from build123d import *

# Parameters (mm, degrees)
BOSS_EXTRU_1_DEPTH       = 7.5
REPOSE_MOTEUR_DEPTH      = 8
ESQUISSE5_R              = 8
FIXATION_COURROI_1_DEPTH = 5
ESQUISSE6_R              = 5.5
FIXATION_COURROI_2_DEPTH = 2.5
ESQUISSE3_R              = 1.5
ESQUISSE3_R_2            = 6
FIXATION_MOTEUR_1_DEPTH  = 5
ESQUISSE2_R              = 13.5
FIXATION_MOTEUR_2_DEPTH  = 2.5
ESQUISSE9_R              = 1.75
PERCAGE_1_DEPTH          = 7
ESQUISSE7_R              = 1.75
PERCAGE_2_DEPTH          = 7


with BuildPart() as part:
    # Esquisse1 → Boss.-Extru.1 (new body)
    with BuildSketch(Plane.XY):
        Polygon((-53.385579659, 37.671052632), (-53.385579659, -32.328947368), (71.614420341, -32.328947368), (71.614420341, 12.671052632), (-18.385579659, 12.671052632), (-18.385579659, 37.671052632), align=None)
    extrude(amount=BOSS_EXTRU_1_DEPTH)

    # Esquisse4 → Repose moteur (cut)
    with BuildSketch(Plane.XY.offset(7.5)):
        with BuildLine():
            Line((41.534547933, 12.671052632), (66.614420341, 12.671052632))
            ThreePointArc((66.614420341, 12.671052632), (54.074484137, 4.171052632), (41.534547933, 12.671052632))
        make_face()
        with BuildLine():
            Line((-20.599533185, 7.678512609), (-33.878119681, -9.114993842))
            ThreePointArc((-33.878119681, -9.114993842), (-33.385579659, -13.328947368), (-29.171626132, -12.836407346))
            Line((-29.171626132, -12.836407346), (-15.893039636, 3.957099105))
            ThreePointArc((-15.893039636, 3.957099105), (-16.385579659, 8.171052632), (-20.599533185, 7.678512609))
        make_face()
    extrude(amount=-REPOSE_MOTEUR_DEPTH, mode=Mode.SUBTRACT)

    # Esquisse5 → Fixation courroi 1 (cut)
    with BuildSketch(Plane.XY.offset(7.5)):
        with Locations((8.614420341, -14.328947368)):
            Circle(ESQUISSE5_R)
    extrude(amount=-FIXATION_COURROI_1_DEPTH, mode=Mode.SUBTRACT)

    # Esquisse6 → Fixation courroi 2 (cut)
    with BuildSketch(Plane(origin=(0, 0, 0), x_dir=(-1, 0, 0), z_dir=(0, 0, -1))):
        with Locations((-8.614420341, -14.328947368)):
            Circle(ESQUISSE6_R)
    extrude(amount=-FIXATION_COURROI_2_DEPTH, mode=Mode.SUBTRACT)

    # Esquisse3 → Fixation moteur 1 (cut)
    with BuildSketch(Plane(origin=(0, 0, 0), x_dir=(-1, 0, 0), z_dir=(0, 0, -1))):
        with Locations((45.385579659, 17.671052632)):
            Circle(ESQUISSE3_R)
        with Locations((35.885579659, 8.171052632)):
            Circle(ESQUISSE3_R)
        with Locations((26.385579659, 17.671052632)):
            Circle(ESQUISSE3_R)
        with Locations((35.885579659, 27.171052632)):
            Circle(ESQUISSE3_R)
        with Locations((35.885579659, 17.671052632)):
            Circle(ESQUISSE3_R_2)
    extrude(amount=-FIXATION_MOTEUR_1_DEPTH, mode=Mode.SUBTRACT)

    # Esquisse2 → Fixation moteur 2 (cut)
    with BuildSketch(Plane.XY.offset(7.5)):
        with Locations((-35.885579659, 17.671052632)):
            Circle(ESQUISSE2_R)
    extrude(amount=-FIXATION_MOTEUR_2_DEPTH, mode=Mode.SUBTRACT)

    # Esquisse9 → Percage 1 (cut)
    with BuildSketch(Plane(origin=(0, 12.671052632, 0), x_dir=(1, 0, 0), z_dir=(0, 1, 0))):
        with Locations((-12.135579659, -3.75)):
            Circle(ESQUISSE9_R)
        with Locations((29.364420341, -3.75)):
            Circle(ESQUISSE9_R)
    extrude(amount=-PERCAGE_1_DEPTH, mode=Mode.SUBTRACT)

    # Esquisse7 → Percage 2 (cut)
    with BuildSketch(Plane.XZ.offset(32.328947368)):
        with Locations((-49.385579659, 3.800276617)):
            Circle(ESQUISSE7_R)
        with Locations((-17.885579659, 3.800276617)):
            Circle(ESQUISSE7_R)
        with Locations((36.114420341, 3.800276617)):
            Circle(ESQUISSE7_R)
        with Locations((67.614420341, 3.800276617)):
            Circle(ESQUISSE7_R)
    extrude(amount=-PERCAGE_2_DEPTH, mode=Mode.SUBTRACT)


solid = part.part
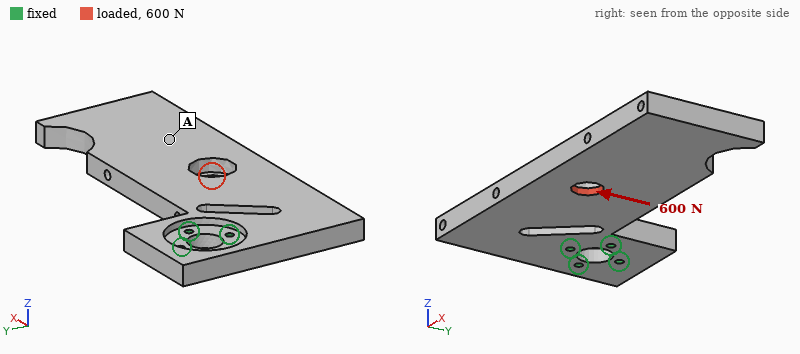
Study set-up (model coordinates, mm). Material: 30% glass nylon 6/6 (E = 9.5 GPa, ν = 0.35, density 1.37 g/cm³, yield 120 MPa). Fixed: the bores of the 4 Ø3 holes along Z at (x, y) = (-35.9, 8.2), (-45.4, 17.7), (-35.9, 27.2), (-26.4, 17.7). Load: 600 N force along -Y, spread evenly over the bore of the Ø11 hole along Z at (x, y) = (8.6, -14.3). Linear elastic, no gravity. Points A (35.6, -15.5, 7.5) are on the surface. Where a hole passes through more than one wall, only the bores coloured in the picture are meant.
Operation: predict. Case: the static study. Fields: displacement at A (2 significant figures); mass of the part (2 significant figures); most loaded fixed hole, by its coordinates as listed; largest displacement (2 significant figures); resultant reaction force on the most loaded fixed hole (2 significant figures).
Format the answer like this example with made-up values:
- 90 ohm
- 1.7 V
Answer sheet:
- 0.35 mm
- 58 g
- (-26.4, 17.7)
- 0.58 mm
- 1.1 kN
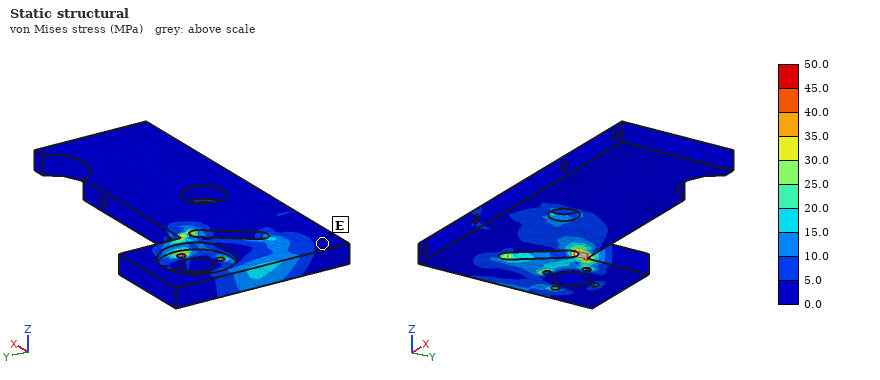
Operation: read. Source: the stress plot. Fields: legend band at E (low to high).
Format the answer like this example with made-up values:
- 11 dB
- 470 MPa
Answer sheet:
- 0.0 to 5.0 MPa
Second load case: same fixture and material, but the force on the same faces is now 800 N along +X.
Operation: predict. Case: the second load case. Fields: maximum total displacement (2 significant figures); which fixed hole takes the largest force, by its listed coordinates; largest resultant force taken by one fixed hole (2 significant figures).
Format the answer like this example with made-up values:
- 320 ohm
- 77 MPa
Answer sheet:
- 1.1 mm
- (-35.9, 8.2)
- 920 N
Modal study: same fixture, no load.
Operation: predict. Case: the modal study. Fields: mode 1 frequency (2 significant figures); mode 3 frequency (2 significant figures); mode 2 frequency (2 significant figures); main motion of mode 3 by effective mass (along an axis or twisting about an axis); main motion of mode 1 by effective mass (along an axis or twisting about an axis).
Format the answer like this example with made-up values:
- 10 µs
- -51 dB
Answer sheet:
- 190 Hz
- 830 Hz
- 790 Hz
- along Y
- along Z
